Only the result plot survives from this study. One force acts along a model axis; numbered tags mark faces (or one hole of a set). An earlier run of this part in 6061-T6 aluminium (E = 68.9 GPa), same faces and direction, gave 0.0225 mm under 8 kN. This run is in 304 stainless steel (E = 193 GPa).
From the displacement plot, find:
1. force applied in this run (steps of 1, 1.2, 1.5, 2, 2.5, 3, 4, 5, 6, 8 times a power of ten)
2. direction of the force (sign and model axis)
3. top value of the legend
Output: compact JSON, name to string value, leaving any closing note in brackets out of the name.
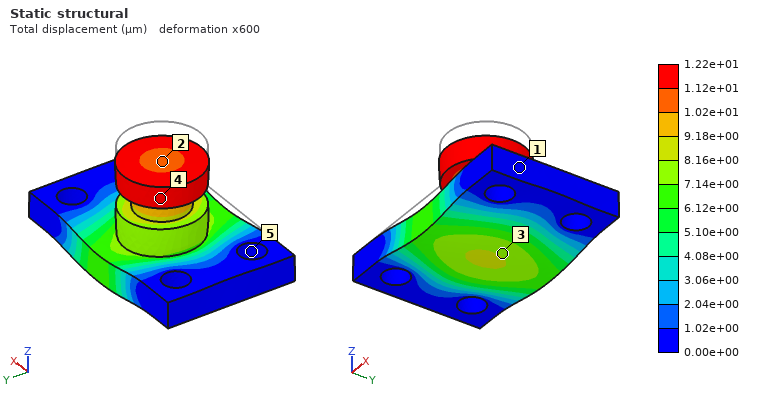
{"force applied in this run": "12 kN", "direction of the force": "-Z", "top value of the legend": "1.22e+01 µm"}
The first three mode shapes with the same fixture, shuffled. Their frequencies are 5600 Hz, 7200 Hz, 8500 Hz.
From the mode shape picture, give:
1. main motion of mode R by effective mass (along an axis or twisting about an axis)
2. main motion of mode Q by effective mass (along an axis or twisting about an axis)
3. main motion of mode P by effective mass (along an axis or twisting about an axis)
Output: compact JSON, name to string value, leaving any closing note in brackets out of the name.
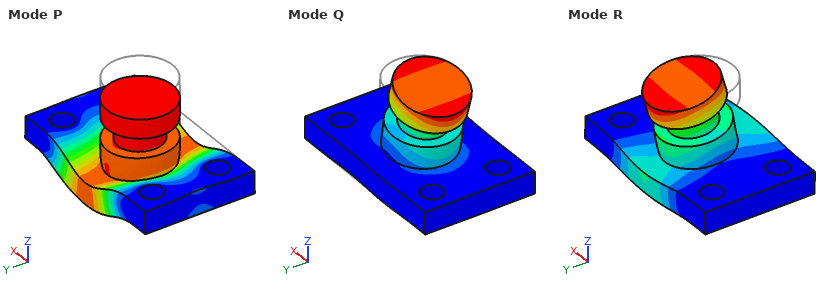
{"main motion of mode R by effective mass": "along Y", "main motion of mode Q by effective mass": "along X", "main motion of mode P by effective mass": "along Z"}
